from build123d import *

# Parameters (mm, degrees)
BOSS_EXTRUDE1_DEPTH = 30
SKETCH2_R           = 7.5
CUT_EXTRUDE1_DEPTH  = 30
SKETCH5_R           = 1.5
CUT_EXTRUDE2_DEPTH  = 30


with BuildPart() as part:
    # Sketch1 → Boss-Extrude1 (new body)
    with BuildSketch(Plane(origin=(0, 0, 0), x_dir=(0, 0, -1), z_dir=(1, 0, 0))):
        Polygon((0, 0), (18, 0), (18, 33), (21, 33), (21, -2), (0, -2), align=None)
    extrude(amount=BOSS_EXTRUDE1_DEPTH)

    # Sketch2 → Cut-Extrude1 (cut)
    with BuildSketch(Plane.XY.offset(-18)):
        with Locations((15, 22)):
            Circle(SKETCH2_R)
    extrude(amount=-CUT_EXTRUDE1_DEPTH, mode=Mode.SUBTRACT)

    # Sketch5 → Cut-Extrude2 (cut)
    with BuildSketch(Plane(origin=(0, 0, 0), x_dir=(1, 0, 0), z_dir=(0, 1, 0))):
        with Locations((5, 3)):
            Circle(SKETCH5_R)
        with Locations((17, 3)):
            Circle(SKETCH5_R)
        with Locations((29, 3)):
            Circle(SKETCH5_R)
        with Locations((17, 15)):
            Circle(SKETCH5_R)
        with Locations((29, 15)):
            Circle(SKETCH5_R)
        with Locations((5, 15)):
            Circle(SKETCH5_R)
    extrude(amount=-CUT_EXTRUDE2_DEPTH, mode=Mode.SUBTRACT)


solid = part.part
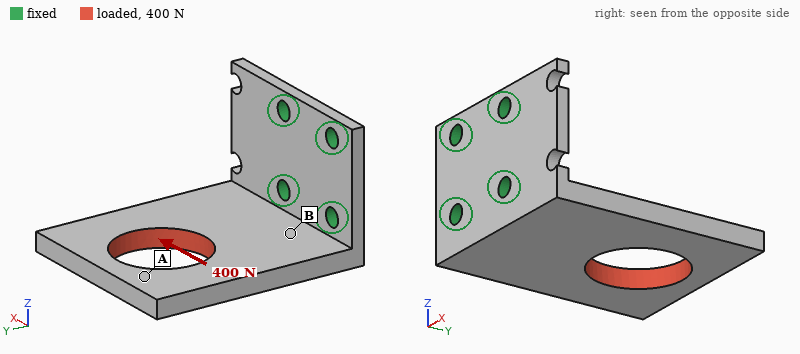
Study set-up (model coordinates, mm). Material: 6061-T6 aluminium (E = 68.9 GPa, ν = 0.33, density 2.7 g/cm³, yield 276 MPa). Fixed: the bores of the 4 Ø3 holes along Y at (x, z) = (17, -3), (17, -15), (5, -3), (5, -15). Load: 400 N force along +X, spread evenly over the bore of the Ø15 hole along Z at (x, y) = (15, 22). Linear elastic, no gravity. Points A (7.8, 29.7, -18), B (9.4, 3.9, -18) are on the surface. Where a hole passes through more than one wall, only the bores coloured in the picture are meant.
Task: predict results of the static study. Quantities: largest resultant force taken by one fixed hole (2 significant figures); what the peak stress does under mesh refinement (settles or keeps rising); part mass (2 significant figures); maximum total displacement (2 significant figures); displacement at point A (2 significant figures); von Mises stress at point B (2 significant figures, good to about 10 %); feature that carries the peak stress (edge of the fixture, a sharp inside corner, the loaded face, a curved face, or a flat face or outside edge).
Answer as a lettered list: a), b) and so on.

a) 700 N
b) keeps rising
c) 9.8 g
d) 0.14 mm
e) 0.10 mm
f) 51 MPa
g) edge of the fixture
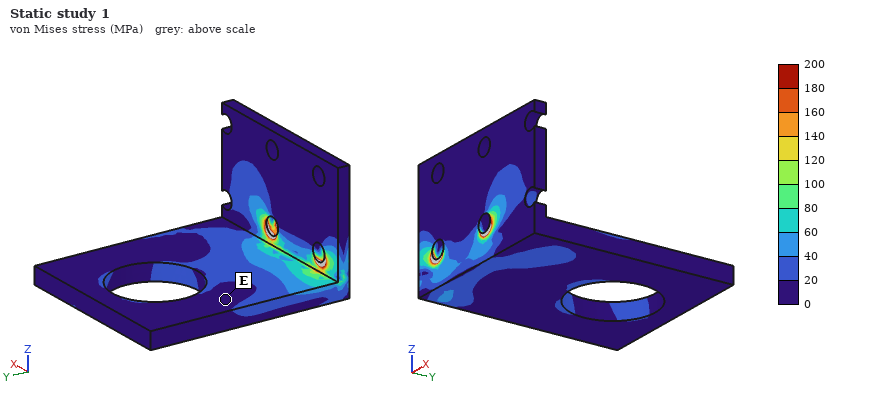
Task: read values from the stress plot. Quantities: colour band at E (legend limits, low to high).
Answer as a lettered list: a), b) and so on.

a) 0 to 20 MPa
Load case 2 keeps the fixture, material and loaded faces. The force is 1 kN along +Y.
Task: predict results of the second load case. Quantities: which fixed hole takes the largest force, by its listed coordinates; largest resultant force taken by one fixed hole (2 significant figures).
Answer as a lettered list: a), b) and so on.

a) (17, -15)
b) 830 N
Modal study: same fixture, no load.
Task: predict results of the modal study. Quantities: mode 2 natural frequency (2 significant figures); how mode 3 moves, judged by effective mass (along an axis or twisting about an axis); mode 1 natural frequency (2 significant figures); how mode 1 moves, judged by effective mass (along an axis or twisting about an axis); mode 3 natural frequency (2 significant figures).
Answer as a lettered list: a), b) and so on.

a) 4100 Hz
b) along X
c) 1500 Hz
d) along Z
e) 5500 Hz
